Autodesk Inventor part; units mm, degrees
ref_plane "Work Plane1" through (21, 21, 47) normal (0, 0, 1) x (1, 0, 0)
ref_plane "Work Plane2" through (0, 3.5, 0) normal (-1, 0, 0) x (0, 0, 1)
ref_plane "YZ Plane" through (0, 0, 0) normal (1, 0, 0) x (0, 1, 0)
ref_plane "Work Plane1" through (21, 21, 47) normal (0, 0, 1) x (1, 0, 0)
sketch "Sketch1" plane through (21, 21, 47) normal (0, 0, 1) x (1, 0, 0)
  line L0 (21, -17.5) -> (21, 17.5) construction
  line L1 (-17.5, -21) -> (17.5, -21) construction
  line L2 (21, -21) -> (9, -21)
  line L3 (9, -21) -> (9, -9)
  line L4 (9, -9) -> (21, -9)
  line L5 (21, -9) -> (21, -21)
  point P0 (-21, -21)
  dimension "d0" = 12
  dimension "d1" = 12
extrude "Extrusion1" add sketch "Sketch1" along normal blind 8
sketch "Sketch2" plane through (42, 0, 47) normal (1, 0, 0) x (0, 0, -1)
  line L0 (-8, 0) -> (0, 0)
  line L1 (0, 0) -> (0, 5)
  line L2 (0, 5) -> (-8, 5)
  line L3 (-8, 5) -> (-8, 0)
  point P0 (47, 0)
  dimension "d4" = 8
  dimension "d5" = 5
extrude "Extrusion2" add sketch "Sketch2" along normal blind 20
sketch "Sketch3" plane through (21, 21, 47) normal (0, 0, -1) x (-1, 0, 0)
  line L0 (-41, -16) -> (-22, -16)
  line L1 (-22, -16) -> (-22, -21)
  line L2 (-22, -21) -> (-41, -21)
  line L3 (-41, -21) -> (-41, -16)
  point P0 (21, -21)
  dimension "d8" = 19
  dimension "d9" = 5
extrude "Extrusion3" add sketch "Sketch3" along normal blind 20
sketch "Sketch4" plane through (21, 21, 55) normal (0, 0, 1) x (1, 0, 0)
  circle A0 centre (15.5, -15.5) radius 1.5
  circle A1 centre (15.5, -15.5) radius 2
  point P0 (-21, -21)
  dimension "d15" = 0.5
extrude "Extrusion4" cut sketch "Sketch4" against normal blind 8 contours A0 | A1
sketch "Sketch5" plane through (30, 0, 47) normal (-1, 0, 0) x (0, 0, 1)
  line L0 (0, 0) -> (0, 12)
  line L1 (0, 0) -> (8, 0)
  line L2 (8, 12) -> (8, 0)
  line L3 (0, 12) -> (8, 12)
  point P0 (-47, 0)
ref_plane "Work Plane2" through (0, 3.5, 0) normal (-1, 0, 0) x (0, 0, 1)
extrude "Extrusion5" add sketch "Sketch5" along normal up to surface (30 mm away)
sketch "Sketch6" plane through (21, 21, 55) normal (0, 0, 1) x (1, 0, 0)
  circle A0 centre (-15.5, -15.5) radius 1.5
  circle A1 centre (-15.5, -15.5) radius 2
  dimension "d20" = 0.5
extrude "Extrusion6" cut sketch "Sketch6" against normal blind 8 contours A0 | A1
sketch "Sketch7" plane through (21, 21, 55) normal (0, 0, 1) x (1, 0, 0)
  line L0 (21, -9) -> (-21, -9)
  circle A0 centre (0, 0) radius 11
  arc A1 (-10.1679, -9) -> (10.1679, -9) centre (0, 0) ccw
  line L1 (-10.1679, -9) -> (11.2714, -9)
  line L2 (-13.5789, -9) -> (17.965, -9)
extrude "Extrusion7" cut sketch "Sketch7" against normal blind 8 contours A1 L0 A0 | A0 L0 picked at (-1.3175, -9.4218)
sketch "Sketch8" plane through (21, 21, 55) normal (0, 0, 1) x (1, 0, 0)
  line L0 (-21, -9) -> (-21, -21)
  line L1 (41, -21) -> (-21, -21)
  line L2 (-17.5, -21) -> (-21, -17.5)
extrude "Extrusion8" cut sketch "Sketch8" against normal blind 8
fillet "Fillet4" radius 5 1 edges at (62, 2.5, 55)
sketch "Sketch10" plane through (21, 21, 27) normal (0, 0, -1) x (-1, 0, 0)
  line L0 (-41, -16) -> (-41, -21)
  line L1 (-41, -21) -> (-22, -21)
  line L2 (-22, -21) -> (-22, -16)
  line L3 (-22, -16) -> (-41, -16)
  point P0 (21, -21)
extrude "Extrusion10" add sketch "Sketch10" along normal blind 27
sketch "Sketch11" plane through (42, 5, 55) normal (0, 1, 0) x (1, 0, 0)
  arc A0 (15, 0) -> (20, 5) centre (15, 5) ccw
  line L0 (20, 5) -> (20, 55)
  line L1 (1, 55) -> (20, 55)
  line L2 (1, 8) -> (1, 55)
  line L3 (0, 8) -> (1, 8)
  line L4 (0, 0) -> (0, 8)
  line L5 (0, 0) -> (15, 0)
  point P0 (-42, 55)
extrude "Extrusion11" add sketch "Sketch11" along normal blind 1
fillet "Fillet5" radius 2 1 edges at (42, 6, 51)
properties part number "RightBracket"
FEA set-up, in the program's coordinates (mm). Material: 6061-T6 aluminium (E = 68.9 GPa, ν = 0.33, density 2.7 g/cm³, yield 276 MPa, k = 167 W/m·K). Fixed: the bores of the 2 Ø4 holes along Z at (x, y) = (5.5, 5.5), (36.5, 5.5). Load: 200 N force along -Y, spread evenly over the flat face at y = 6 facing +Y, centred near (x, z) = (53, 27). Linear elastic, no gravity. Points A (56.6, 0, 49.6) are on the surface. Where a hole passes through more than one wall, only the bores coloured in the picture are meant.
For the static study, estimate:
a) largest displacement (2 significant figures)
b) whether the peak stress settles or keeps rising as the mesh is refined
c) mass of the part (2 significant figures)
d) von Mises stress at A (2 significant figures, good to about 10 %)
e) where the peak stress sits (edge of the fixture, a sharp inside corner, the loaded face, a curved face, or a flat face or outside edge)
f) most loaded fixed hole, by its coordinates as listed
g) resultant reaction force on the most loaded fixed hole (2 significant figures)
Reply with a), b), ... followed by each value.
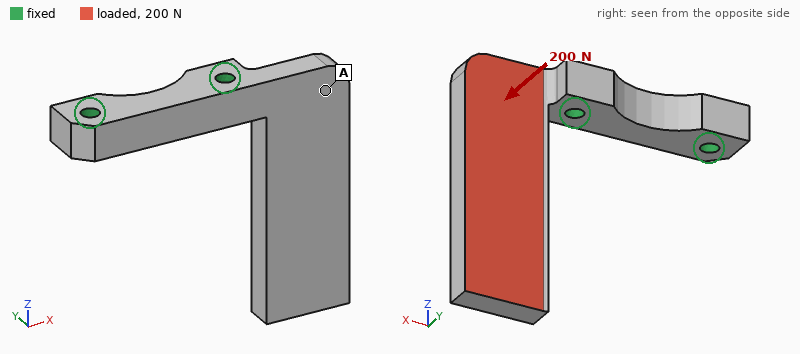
a) 0.33 mm
b) keeps rising
c) 26 g
d) 18 MPa
e) a sharp inside corner
f) (36.5, 5.5)
g) 240 N
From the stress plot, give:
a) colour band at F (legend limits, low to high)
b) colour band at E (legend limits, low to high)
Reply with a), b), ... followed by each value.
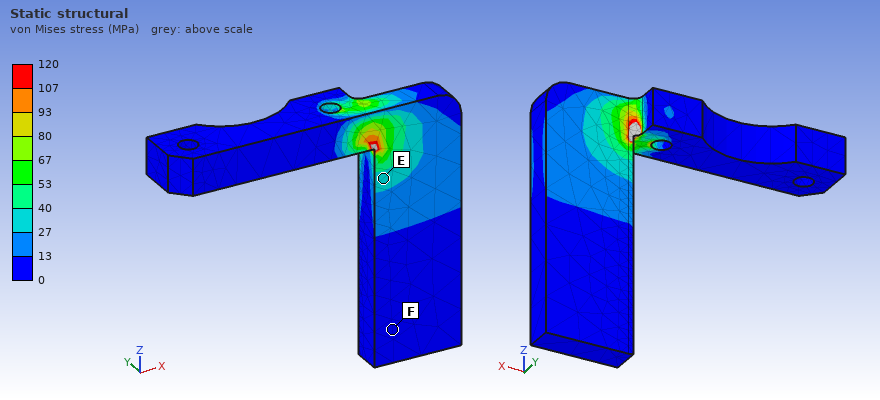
a) 0 to 13 MPa
b) 27 to 40 MPa
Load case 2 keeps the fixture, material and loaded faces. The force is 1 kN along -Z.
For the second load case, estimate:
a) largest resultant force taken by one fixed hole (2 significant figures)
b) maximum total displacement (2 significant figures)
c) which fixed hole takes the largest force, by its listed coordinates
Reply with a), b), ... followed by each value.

a) 1.0 kN
b) 0.39 mm
c) (36.5, 5.5)
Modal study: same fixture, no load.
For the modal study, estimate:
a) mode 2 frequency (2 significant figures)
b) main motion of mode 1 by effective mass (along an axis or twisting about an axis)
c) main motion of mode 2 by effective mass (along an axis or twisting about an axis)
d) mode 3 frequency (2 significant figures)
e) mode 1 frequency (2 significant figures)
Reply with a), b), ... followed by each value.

a) 1700 Hz
b) along Y
c) along X
d) 4700 Hz
e) 1200 Hz
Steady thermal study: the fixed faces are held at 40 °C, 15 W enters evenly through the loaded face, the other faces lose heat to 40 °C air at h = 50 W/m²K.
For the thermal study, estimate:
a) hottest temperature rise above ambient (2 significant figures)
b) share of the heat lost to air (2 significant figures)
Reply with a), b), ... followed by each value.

a) 29 K
b) 15 %
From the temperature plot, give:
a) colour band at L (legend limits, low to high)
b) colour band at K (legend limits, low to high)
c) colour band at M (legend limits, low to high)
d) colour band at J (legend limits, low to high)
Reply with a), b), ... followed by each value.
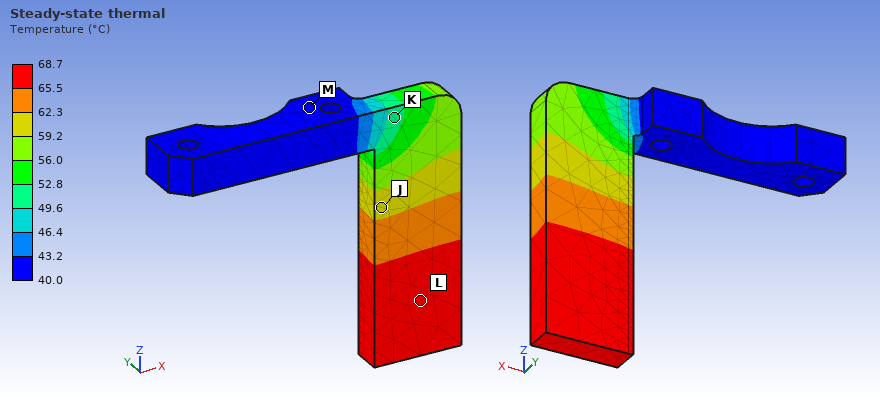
a) 65.5 to 68.7 °C
b) 49.6 to 52.8 °C
c) 40.0 to 43.2 °C
d) 59.2 to 62.3 °C
